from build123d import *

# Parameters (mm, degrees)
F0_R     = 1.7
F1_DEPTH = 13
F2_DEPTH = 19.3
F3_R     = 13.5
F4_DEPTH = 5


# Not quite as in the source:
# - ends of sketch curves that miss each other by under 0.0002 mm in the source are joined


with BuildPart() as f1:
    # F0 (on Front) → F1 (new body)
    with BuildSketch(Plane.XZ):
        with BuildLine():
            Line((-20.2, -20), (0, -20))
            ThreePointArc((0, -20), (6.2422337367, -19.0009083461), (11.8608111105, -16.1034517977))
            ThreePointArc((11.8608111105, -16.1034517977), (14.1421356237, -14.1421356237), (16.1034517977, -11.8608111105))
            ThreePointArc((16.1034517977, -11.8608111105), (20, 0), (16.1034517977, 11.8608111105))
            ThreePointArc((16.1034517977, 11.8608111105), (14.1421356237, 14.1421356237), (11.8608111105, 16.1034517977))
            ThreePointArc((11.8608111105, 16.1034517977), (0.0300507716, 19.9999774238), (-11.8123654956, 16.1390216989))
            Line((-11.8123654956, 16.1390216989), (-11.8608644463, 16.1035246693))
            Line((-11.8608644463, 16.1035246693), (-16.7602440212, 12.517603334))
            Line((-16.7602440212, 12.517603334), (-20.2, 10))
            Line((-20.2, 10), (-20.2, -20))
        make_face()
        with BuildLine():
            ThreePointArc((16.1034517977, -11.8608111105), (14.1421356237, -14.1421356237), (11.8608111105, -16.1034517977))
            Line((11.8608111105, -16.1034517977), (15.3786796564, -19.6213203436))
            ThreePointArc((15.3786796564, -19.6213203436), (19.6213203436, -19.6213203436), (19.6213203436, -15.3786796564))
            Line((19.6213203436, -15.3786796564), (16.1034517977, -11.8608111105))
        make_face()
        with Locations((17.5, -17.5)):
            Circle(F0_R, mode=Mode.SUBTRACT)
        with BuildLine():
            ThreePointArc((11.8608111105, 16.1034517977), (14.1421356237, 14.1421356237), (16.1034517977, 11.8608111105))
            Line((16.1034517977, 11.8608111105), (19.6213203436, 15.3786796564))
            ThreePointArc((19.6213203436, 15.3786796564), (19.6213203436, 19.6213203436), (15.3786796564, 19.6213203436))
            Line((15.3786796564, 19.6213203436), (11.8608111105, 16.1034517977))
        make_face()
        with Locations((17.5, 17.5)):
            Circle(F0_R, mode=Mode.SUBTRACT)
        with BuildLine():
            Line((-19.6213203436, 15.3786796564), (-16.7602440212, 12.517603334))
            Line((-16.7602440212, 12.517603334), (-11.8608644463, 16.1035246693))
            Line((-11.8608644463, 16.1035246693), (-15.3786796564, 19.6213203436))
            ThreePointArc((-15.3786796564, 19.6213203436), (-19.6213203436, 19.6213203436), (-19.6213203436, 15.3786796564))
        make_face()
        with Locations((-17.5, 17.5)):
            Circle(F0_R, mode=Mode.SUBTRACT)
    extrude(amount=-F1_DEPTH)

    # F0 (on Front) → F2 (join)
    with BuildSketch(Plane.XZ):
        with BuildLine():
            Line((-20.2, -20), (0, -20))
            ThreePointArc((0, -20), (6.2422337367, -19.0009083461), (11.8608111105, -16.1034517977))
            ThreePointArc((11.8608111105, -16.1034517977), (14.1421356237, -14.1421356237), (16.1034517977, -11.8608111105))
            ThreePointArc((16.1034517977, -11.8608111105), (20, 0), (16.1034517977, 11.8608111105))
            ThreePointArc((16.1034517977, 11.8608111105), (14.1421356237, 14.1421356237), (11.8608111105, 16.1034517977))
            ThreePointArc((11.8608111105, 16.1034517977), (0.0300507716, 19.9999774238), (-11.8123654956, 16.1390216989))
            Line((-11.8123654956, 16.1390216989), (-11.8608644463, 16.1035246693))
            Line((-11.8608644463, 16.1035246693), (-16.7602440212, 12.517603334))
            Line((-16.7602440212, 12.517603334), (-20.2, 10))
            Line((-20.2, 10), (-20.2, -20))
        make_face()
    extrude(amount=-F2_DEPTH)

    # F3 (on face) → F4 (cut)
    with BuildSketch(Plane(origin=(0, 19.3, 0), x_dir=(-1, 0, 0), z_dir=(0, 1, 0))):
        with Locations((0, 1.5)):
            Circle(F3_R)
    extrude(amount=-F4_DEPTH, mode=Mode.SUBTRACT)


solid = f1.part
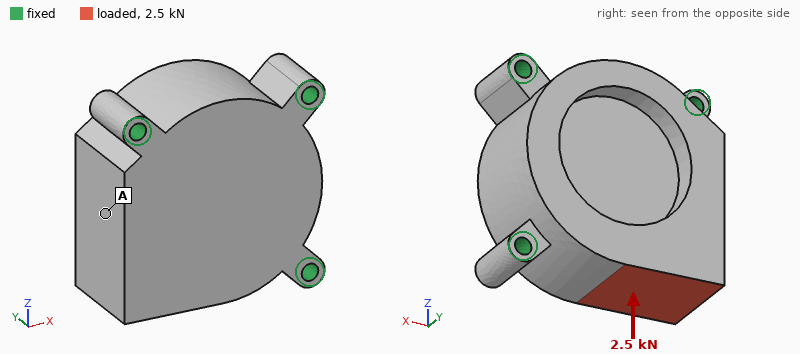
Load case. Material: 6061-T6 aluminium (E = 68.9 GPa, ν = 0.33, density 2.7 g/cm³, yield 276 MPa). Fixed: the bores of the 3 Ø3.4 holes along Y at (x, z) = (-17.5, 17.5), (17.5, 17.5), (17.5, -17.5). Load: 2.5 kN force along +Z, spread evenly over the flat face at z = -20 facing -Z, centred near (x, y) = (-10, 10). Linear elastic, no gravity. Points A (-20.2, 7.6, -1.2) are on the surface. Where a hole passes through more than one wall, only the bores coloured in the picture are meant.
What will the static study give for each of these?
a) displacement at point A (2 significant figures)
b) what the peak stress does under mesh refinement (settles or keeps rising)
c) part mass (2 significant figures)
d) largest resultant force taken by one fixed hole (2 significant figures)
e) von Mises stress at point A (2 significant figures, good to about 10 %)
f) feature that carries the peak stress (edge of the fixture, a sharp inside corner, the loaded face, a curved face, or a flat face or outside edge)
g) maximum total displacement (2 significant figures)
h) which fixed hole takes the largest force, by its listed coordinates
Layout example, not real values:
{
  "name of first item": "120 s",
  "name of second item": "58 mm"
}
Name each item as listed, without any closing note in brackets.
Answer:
{
  "displacement at point A": "5.4 µm",
  "what the peak stress does under mesh refinement": "keeps rising",
  "part mass": "67 g",
  "largest resultant force taken by one fixed hole": "1.5 kN",
  "von Mises stress at point A": "8.0 MPa",
  "feature that carries the peak stress": "edge of the fixture",
  "maximum total displacement": "11 µm",
  "which fixed hole takes the largest force, by its listed coordinates": "(-17.5, 17.5)"
}
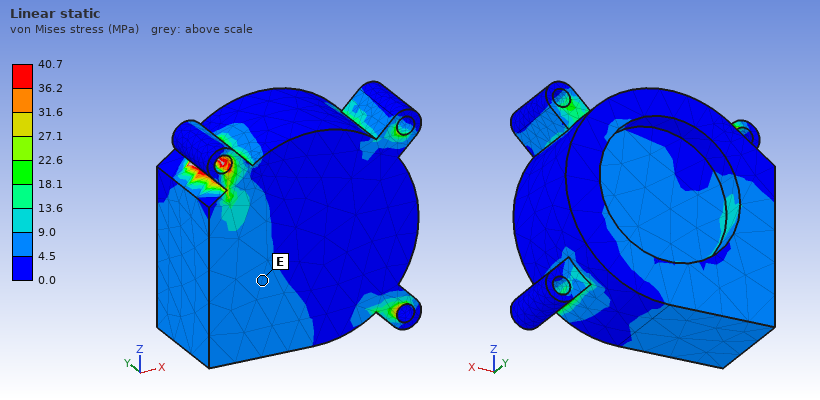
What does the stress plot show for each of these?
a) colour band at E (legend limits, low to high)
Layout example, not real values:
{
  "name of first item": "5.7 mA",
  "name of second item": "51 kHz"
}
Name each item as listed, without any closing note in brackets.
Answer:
{
  "colour band at E": "4.5 to 9.0 MPa"
}
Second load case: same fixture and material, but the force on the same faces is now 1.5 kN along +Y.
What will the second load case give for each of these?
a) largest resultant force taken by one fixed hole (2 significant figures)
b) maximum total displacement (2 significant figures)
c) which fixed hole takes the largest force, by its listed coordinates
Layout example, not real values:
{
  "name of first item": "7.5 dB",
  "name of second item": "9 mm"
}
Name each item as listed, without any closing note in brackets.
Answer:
{
  "largest resultant force taken by one fixed hole": "1.4 kN",
  "maximum total displacement": "53 µm",
  "which fixed hole takes the largest force, by its listed coordinates": "(17.5, -17.5)"
}
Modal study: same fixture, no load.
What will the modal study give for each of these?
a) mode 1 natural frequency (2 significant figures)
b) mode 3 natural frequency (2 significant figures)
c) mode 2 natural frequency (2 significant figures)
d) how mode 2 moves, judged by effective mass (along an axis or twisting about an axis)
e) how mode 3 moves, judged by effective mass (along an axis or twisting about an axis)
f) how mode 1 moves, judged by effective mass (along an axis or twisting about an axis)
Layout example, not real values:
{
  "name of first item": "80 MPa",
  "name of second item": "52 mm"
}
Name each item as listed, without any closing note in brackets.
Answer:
{
  "mode 1 natural frequency": "8100 Hz",
  "mode 3 natural frequency": "20 kHz",
  "mode 2 natural frequency": "19 kHz",
  "how mode 2 moves, judged by effective mass": "along X",
  "how mode 3 moves, judged by effective mass": "along Z",
  "how mode 1 moves, judged by effective mass": "along Y"
}
